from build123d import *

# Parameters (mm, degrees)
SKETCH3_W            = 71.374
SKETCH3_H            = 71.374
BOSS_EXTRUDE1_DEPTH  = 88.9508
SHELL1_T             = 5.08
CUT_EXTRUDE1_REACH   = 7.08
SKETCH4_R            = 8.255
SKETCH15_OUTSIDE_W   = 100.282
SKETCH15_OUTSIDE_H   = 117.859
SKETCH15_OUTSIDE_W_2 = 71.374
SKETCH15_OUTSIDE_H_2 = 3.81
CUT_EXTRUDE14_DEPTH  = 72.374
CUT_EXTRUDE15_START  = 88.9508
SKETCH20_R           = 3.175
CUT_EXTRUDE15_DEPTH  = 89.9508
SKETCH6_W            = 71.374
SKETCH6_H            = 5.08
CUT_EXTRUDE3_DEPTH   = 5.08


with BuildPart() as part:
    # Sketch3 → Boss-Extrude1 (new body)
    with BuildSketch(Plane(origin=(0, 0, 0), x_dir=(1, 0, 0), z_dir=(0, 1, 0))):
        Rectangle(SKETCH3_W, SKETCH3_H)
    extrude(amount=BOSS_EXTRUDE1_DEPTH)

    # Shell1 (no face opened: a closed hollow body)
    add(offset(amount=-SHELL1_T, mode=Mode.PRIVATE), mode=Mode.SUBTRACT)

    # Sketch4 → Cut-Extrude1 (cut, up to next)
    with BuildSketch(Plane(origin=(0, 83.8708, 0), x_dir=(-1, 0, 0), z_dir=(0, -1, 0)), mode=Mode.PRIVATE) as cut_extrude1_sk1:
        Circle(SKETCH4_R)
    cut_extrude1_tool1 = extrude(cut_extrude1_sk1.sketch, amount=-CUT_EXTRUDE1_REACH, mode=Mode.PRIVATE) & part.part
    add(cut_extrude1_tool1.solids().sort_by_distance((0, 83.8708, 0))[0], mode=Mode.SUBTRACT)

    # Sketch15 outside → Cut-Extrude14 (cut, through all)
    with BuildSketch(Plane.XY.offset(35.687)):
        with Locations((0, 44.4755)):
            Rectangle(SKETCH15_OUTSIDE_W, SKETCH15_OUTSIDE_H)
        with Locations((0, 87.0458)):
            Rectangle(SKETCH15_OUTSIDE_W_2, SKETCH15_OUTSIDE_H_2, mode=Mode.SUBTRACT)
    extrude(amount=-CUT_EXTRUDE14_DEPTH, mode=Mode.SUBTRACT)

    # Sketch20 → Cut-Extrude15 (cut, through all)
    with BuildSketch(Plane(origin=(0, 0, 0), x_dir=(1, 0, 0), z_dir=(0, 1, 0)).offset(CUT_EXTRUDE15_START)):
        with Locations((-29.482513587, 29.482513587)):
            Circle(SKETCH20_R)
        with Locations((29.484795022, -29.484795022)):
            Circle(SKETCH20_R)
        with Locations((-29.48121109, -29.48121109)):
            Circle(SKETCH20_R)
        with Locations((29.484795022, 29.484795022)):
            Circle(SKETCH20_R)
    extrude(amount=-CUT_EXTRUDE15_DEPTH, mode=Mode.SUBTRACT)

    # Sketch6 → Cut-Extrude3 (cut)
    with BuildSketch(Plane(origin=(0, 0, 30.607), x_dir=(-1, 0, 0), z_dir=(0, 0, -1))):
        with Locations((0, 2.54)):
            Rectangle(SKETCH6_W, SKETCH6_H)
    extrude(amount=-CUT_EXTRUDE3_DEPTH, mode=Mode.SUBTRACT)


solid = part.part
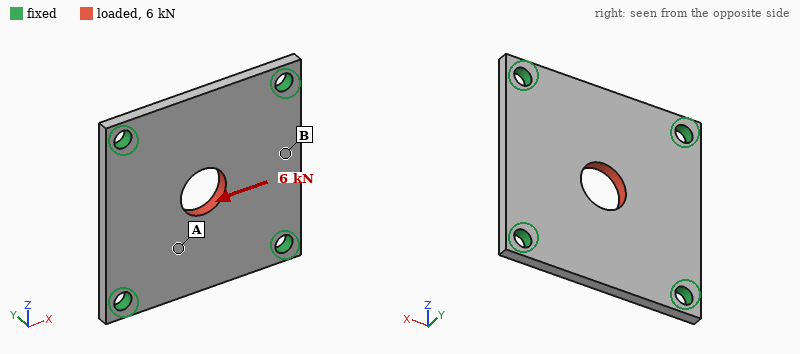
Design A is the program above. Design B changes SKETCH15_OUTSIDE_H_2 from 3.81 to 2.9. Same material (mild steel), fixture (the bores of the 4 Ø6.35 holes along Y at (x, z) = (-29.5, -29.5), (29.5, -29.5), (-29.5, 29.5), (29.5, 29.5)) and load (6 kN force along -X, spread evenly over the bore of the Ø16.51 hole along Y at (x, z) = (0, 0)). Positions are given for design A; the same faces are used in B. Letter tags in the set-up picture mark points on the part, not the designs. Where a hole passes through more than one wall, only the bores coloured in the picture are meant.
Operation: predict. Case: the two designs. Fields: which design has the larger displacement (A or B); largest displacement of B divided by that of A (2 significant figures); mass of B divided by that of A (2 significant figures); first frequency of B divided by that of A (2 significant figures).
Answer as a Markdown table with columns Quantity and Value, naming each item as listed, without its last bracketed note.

| Quantity | Value |
|---|---|
| which design has the larger displacement | B |
| largest displacement of B divided by that of A | 1.3 |
| mass of B divided by that of A | 0.76 |
| first frequency of B divided by that of A | 0.78 |
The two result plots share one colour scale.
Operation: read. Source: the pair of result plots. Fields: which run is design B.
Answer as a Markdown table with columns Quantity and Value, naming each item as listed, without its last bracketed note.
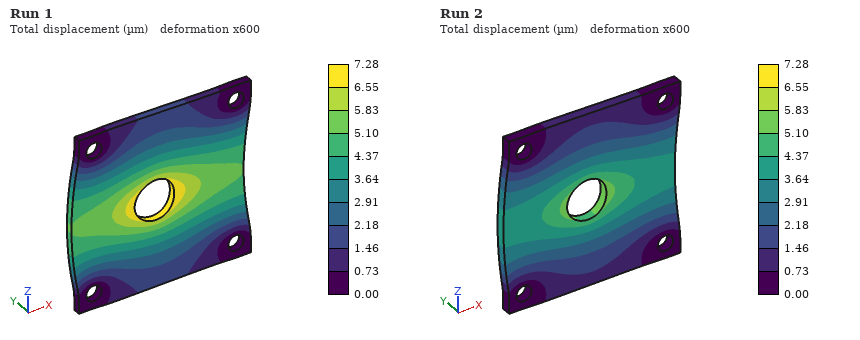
| Quantity | Value |
|---|---|
| which run is design B | Run 1 |
